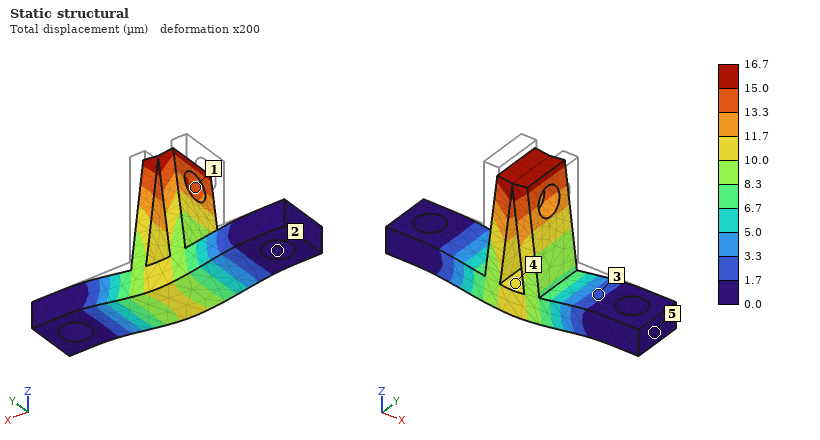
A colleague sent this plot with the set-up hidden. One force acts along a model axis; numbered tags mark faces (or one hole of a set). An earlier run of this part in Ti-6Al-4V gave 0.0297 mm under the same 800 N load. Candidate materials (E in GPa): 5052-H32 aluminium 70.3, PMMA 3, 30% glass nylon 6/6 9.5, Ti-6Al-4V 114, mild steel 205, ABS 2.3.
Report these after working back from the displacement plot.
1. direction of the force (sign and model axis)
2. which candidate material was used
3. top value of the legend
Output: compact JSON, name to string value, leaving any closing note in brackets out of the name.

{"direction of the force": "-Z", "which candidate material was used": "mild steel", "top value of the legend": "16.7 µm"}
